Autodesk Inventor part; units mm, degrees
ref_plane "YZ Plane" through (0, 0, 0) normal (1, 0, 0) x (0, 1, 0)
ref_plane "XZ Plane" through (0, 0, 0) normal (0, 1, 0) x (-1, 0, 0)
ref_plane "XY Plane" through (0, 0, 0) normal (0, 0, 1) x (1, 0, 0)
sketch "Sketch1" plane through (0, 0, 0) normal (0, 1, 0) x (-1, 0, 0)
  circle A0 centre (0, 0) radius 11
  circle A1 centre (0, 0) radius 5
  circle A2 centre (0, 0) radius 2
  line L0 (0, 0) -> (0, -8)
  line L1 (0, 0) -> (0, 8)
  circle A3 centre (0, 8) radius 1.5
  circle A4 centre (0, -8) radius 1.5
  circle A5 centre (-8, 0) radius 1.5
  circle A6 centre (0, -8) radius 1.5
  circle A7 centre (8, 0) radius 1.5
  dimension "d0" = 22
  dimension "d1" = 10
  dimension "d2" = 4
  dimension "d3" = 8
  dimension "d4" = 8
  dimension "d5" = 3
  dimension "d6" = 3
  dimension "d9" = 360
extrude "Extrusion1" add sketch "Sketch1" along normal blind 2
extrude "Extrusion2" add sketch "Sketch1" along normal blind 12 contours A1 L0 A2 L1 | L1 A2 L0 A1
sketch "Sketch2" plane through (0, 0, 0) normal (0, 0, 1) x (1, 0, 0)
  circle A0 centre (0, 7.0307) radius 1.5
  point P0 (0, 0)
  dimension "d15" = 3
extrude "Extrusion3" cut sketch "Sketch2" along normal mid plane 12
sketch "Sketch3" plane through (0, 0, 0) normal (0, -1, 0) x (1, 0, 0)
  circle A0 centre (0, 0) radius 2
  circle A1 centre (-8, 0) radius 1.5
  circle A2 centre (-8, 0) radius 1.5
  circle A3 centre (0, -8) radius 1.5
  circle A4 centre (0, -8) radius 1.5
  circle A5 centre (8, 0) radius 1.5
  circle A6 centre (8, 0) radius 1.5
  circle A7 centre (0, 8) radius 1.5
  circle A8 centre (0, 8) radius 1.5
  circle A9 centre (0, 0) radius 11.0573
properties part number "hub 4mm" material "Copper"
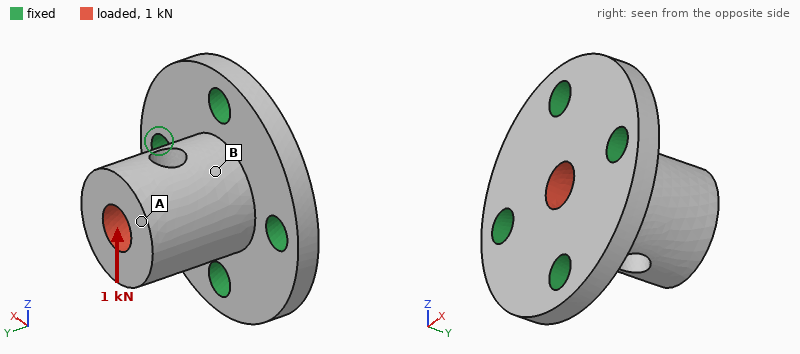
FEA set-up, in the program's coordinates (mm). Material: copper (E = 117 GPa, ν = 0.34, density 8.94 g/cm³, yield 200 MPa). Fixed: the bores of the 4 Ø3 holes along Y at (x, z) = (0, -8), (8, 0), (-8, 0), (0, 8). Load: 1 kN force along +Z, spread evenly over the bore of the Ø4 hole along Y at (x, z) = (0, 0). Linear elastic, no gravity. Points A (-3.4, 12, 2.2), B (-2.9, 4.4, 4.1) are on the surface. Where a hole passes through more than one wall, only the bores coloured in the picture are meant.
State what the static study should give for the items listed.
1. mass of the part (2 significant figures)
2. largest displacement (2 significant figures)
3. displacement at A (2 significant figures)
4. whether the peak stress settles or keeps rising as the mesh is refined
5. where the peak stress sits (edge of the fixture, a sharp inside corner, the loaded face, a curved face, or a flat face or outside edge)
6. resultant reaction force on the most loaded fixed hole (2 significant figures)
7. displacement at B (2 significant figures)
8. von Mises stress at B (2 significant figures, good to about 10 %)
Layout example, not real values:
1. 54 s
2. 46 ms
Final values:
1. 12 g
2. 12 µm
3. 11 µm
4. keeps rising
5. edge of the fixture
6. 510 N
7. 4.6 µm
8. 31 MPa
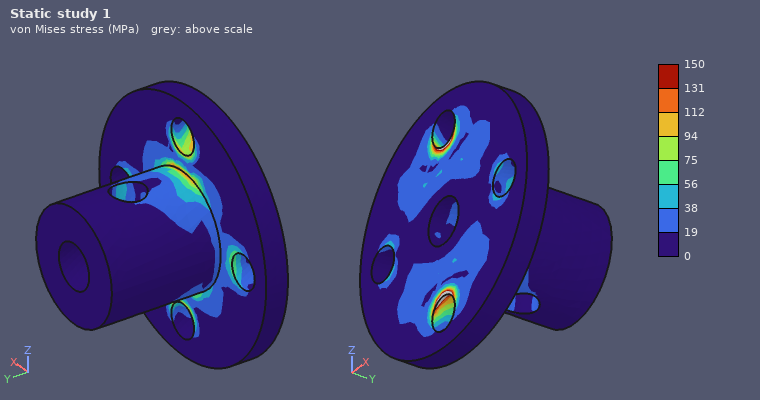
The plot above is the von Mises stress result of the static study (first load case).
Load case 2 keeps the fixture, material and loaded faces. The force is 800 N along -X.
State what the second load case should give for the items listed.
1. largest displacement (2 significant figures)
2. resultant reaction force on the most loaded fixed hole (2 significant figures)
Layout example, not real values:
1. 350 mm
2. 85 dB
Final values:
1. 10 µm
2. 400 N
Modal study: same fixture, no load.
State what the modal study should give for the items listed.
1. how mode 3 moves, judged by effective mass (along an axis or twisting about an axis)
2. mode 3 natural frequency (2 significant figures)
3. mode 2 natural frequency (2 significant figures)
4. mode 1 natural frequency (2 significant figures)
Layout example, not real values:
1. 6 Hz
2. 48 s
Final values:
1. along Y
2. 35 kHz
3. 21 kHz
4. 20 kHz
